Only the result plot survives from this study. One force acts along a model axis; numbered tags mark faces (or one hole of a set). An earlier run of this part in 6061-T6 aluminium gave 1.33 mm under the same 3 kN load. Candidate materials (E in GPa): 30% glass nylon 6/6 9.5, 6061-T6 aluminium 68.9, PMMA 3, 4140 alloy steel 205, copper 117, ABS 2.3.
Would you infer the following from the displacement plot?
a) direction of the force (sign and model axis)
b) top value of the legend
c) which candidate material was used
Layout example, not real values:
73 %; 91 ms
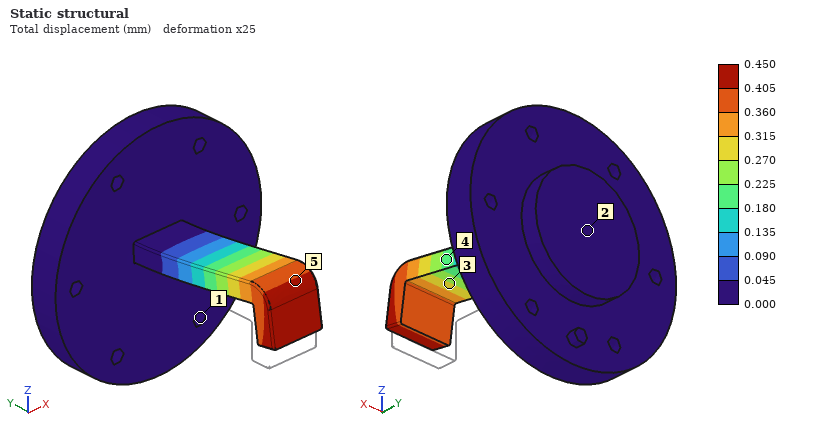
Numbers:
+Z; 0.450 mm; 4140 alloy steel
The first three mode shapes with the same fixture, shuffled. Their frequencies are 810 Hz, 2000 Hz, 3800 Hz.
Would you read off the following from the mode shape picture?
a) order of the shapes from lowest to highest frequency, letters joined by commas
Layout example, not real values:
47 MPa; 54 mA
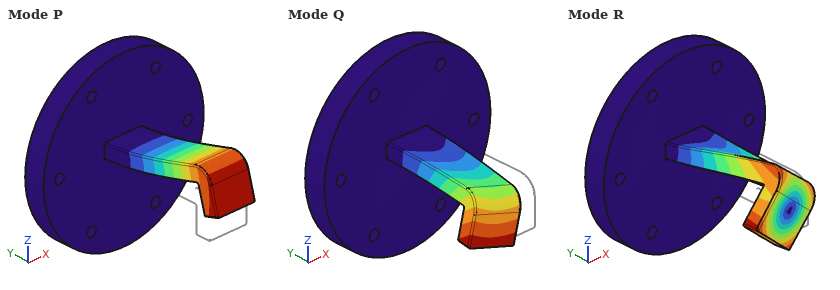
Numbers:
P, Q, R
